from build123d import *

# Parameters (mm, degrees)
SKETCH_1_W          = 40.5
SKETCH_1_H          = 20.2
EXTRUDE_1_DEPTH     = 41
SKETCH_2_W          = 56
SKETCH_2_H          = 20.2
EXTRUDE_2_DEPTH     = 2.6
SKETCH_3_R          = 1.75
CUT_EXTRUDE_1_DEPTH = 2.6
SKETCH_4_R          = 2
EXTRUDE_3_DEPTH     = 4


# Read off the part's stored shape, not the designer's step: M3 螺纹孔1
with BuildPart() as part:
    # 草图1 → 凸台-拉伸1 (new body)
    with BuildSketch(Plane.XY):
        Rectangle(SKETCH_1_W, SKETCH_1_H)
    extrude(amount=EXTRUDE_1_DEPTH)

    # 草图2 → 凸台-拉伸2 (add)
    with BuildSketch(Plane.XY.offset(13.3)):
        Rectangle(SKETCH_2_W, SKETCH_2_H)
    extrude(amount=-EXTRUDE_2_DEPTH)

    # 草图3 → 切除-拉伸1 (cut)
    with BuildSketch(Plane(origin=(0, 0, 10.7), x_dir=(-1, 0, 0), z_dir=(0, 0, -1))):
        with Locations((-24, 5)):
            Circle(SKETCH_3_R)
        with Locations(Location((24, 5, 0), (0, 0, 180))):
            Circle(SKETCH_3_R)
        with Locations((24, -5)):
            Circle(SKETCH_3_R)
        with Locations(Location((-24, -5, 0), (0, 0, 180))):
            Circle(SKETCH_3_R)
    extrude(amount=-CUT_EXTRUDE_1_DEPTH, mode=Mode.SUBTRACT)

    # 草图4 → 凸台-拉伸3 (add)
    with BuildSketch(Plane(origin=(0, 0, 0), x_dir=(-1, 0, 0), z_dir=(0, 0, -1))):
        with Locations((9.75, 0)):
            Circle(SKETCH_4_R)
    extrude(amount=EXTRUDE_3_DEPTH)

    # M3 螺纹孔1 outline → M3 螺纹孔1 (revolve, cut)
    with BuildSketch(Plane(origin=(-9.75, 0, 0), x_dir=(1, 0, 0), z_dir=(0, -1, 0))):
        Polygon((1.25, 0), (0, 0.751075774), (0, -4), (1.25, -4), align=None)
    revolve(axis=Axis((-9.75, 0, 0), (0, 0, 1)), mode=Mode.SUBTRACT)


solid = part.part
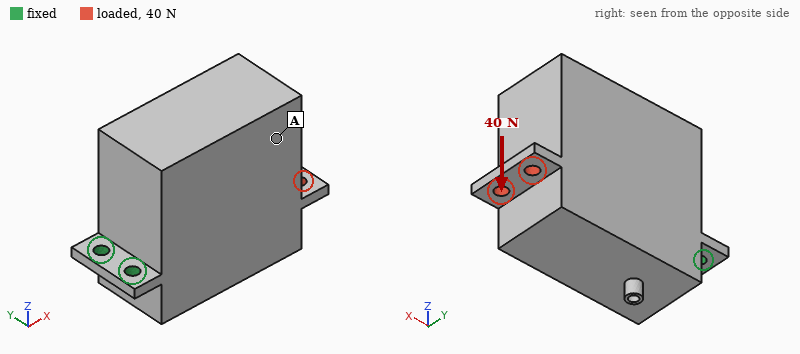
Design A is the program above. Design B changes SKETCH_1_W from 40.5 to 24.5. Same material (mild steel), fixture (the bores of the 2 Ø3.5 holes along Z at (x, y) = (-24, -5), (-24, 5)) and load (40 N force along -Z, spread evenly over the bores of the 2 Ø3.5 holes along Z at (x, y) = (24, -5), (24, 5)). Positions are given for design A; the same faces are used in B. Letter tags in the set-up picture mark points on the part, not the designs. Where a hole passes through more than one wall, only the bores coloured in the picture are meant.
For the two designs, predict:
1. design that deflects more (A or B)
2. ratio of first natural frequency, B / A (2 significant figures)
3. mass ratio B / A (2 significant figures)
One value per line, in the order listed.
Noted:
B
0.85
0.64
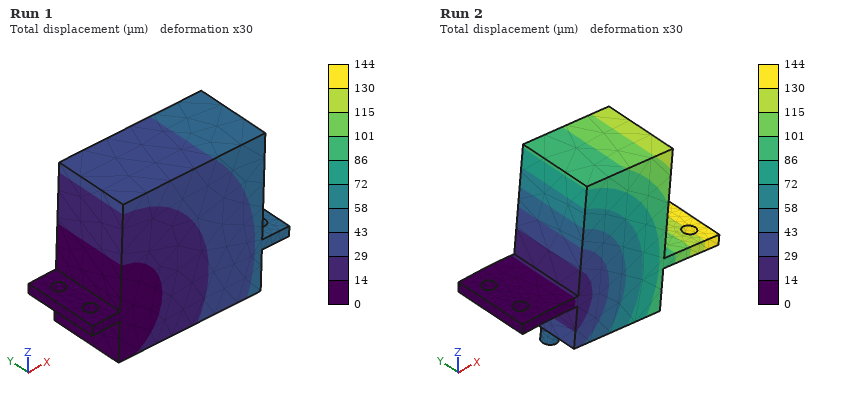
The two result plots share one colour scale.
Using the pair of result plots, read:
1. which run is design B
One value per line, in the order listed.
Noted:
Run 2
